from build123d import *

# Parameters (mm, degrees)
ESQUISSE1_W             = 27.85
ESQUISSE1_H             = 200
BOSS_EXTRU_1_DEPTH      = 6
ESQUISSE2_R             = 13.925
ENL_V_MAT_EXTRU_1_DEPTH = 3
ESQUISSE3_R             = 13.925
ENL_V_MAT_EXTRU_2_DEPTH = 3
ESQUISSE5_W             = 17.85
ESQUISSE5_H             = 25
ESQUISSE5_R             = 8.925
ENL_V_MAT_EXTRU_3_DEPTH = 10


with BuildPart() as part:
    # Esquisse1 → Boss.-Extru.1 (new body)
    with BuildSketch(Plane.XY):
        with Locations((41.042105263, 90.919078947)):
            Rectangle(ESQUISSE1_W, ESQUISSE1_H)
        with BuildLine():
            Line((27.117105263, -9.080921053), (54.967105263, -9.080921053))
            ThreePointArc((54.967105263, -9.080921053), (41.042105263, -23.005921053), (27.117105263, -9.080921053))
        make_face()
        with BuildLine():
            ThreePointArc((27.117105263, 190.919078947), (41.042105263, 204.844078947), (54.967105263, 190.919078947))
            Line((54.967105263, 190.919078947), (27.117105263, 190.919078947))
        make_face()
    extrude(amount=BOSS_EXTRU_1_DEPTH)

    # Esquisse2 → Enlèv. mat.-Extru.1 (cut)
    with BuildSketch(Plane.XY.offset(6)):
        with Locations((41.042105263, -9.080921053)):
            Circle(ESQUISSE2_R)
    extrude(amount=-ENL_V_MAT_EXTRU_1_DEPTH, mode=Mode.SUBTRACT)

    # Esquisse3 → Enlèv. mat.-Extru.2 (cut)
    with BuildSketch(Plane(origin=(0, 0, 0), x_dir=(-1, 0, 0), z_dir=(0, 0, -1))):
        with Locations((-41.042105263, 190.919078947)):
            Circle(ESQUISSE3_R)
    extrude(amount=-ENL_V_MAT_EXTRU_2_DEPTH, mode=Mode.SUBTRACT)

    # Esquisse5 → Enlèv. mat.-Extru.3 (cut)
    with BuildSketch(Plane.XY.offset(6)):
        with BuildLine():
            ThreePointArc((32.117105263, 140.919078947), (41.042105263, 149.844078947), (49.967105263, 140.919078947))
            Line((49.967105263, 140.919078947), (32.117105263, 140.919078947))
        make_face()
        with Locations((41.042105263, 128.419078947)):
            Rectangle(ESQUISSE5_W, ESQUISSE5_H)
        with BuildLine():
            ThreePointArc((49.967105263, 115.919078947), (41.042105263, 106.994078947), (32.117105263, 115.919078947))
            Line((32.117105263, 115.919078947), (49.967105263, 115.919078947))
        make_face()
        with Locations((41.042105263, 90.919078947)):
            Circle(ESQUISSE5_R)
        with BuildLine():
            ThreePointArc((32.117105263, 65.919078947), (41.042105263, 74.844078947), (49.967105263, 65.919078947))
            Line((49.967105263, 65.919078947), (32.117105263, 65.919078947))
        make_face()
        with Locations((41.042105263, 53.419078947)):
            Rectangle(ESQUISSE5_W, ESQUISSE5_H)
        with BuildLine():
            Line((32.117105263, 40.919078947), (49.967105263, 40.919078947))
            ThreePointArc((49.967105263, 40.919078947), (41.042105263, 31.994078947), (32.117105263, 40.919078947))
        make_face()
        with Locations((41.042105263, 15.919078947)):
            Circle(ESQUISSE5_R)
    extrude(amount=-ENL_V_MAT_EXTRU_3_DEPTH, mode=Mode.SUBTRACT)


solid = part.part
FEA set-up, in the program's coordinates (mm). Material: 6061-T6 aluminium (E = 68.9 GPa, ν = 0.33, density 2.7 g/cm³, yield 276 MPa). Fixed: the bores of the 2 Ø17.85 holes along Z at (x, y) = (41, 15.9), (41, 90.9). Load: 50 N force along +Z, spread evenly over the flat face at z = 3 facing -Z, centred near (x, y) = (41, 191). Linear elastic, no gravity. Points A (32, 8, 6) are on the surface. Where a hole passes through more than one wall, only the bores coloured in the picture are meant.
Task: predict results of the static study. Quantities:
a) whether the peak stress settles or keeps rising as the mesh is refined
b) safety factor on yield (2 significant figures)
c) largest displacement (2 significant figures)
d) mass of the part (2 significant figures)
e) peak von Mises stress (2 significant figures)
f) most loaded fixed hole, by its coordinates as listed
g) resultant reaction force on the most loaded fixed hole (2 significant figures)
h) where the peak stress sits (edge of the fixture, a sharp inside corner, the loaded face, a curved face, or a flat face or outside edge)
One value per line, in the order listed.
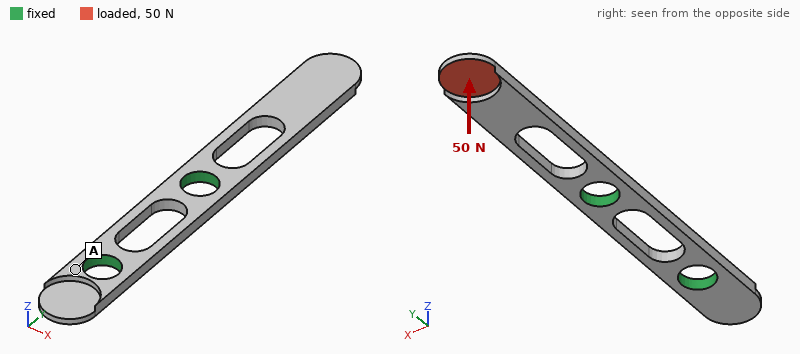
settles
3.8
1.0 mm
60 g
73 MPa
(41, 90.9)
50 N
a curved face
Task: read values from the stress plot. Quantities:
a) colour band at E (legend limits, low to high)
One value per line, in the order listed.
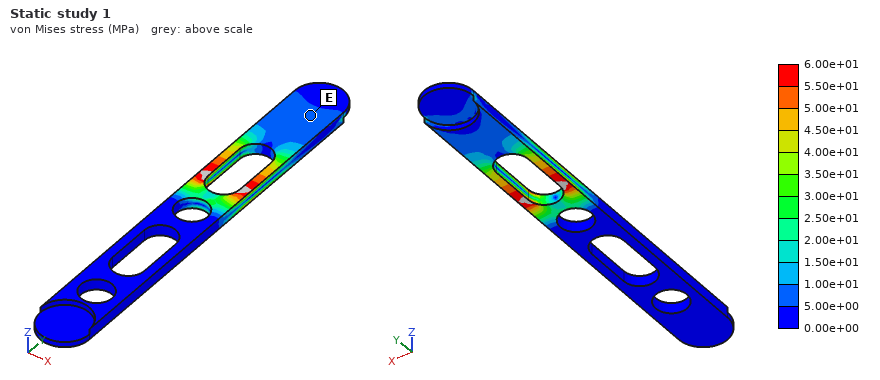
5.00e+00 to 1.00e+01 MPa
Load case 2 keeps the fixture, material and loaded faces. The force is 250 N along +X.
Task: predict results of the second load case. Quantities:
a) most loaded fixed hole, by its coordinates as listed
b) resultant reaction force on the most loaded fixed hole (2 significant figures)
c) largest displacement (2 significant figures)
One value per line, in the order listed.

(41, 90.9)
250 N
0.30 mm
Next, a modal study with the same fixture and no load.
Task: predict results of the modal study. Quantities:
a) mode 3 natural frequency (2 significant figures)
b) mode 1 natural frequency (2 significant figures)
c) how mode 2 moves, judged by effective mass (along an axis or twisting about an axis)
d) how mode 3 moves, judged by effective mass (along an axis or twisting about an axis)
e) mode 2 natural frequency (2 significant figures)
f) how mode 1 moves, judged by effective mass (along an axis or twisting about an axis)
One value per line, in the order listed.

2100 Hz
380 Hz
along X
twisting about Y
1200 Hz
along Z
